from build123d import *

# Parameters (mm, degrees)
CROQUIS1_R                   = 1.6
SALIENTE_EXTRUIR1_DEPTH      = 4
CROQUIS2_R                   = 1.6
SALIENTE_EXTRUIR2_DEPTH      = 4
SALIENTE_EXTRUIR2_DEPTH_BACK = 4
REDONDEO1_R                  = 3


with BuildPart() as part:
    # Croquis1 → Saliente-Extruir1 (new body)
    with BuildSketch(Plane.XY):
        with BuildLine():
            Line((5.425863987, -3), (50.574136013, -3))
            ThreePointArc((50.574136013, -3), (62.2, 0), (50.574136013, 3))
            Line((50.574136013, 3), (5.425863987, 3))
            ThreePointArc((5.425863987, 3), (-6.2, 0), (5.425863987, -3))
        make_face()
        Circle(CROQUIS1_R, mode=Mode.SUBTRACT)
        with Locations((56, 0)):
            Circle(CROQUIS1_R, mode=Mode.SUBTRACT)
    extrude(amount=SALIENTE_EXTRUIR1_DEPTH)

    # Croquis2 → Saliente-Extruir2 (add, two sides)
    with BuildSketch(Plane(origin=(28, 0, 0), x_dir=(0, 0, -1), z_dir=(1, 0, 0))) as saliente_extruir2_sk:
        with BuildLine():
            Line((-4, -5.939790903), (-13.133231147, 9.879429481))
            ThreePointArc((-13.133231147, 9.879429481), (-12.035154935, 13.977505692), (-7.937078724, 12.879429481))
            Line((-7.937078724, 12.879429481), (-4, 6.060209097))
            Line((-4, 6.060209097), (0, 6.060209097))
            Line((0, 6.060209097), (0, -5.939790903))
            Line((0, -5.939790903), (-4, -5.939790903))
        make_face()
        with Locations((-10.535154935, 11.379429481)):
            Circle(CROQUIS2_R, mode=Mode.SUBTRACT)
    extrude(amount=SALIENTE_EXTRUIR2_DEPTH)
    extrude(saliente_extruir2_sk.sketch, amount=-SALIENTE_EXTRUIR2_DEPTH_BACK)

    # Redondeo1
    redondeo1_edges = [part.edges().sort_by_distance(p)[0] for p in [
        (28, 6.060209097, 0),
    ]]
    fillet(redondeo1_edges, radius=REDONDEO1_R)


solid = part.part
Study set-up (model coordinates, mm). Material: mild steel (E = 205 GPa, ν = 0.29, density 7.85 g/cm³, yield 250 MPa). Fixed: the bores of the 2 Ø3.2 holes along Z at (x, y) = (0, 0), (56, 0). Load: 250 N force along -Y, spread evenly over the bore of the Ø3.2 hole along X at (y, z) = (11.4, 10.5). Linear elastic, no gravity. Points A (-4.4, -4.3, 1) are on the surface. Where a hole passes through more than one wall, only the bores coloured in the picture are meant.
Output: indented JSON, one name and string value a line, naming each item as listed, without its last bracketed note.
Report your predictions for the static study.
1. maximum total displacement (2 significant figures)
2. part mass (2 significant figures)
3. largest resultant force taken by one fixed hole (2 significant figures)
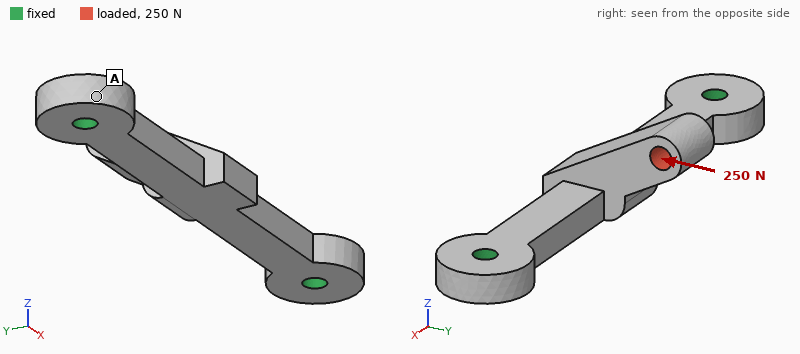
{
  "maximum total displacement": "78 µm",
  "part mass": "22 g",
  "largest resultant force taken by one fixed hole": "130 N"
}
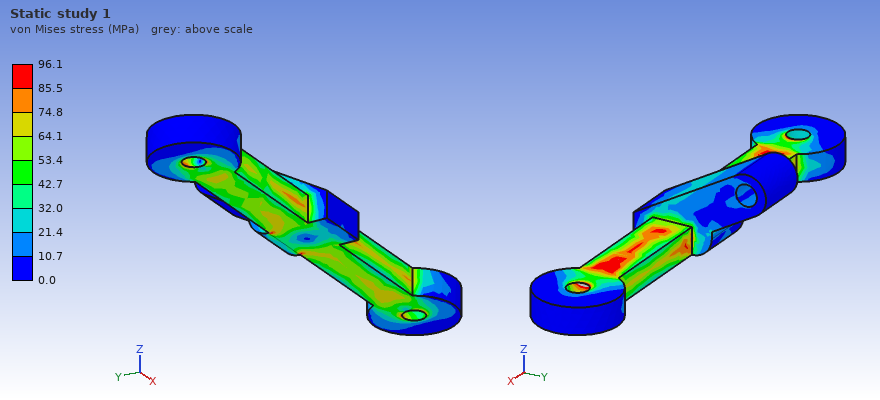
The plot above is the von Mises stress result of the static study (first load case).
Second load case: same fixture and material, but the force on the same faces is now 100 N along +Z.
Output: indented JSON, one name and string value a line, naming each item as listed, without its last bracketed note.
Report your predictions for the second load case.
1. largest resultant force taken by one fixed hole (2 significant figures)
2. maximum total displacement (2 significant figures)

{
  "largest resultant force taken by one fixed hole": "52 N",
  "maximum total displacement": "46 µm"
}
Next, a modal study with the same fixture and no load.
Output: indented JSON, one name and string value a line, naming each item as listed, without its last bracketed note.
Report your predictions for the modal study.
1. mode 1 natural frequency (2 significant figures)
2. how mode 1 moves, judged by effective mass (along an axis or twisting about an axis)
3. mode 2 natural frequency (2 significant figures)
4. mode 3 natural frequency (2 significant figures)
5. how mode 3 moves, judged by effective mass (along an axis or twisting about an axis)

{
  "mode 1 natural frequency": "4100 Hz",
  "how mode 1 moves, judged by effective mass": "along Z",
  "mode 2 natural frequency": "5800 Hz",
  "mode 3 natural frequency": "8900 Hz",
  "how mode 3 moves, judged by effective mass": "along Y"
}
